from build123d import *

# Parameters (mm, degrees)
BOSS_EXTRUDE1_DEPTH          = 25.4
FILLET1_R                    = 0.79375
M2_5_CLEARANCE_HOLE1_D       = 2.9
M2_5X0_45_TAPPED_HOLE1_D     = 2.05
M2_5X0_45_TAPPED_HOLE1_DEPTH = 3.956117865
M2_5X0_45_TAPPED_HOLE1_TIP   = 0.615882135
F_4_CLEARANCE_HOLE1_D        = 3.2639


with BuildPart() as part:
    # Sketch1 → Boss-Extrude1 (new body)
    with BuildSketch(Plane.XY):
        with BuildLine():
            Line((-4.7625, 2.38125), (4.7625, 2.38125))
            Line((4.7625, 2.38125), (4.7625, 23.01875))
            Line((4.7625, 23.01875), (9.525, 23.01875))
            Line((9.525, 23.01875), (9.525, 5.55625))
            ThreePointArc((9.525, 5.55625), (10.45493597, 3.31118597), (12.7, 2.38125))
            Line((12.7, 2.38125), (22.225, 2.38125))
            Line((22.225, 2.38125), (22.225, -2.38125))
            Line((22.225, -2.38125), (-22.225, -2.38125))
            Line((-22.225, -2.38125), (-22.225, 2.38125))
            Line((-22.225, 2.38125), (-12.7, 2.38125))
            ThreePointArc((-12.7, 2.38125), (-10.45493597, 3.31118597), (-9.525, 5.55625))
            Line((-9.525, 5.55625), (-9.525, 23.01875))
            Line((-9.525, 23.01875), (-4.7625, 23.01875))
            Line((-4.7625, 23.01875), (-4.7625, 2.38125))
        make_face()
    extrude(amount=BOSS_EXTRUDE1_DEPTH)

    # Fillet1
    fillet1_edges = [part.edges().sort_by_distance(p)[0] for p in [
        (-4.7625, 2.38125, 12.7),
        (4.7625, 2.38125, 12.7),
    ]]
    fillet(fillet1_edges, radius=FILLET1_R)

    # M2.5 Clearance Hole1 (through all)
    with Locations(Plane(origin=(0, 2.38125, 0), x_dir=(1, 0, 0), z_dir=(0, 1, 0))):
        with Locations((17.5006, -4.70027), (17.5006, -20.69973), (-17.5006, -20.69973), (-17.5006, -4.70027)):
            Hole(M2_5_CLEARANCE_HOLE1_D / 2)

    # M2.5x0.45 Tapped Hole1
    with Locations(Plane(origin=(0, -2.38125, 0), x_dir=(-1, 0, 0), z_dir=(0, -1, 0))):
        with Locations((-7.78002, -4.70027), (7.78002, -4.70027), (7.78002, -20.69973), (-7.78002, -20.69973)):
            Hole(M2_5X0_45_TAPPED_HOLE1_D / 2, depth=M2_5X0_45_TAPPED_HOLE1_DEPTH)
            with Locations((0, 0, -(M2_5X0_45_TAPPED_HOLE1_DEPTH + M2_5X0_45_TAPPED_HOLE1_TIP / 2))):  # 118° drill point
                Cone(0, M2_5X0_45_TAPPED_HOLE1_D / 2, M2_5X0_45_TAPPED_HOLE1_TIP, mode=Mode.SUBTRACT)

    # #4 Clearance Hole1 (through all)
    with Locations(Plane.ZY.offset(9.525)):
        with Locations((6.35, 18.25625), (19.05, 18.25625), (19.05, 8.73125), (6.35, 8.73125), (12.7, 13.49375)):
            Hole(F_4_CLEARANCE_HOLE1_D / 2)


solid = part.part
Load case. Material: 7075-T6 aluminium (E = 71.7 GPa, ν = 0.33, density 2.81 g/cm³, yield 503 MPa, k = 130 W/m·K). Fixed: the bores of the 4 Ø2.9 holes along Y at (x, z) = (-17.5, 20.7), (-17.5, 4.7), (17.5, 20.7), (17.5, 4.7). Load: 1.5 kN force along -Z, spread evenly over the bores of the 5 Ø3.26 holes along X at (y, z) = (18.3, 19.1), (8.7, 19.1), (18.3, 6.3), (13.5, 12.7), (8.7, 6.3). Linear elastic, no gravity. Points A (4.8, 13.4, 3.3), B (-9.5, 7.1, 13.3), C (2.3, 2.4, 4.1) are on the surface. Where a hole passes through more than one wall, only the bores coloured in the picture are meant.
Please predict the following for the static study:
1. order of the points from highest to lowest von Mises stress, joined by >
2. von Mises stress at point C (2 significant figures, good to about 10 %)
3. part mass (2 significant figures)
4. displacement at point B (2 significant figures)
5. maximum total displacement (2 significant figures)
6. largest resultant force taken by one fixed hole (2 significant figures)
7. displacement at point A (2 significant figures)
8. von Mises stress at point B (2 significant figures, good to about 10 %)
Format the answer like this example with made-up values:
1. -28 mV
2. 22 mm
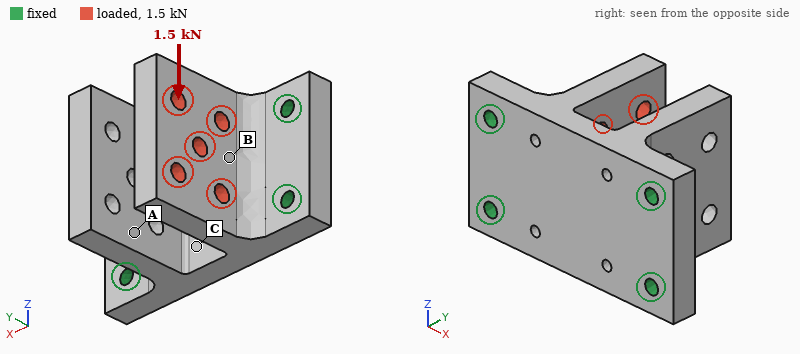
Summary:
1. B > C > A
2. 28 MPa
3. 28 g
4. 18 µm
5. 60 µm
6. 1.1 kN
7. 13 µm
8. 48 MPa
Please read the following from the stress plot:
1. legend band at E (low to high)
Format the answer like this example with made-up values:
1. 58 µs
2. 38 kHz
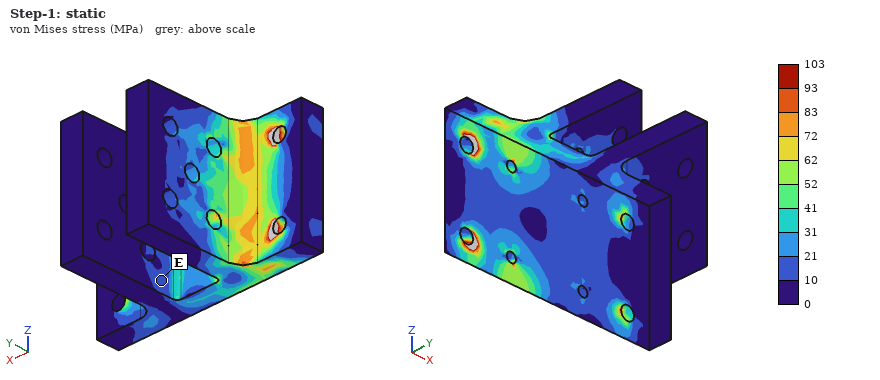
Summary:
1. 10 to 21 MPa
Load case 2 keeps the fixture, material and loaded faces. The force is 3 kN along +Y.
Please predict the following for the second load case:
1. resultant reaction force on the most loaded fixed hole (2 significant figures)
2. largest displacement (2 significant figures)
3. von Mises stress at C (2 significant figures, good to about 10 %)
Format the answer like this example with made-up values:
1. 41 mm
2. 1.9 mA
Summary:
1. 1.1 kN
2. 66 µm
3. 42 MPa
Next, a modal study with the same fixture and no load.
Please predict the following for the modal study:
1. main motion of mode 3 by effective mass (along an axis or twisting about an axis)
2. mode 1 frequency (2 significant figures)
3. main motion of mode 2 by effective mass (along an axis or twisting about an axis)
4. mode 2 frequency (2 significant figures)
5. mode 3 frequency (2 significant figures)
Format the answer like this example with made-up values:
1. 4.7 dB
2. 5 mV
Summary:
1. along Z
2. 6200 Hz
3. along X
4. 8100 Hz
5. 9600 Hz
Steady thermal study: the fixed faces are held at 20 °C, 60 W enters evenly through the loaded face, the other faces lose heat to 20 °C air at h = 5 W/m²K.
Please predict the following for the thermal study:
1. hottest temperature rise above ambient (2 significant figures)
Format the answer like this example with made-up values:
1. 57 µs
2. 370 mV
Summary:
1. 78 K
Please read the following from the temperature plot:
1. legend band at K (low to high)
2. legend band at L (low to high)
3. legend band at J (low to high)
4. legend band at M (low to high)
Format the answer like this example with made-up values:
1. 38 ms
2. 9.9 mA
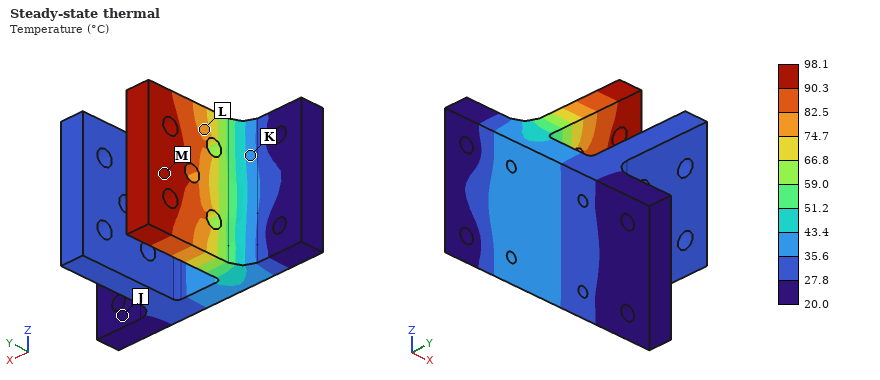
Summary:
1. 35.6 to 43.4 °C
2. 74.7 to 82.5 °C
3. 20.0 to 27.8 °C
4. 90.3 to 98.1 °C
